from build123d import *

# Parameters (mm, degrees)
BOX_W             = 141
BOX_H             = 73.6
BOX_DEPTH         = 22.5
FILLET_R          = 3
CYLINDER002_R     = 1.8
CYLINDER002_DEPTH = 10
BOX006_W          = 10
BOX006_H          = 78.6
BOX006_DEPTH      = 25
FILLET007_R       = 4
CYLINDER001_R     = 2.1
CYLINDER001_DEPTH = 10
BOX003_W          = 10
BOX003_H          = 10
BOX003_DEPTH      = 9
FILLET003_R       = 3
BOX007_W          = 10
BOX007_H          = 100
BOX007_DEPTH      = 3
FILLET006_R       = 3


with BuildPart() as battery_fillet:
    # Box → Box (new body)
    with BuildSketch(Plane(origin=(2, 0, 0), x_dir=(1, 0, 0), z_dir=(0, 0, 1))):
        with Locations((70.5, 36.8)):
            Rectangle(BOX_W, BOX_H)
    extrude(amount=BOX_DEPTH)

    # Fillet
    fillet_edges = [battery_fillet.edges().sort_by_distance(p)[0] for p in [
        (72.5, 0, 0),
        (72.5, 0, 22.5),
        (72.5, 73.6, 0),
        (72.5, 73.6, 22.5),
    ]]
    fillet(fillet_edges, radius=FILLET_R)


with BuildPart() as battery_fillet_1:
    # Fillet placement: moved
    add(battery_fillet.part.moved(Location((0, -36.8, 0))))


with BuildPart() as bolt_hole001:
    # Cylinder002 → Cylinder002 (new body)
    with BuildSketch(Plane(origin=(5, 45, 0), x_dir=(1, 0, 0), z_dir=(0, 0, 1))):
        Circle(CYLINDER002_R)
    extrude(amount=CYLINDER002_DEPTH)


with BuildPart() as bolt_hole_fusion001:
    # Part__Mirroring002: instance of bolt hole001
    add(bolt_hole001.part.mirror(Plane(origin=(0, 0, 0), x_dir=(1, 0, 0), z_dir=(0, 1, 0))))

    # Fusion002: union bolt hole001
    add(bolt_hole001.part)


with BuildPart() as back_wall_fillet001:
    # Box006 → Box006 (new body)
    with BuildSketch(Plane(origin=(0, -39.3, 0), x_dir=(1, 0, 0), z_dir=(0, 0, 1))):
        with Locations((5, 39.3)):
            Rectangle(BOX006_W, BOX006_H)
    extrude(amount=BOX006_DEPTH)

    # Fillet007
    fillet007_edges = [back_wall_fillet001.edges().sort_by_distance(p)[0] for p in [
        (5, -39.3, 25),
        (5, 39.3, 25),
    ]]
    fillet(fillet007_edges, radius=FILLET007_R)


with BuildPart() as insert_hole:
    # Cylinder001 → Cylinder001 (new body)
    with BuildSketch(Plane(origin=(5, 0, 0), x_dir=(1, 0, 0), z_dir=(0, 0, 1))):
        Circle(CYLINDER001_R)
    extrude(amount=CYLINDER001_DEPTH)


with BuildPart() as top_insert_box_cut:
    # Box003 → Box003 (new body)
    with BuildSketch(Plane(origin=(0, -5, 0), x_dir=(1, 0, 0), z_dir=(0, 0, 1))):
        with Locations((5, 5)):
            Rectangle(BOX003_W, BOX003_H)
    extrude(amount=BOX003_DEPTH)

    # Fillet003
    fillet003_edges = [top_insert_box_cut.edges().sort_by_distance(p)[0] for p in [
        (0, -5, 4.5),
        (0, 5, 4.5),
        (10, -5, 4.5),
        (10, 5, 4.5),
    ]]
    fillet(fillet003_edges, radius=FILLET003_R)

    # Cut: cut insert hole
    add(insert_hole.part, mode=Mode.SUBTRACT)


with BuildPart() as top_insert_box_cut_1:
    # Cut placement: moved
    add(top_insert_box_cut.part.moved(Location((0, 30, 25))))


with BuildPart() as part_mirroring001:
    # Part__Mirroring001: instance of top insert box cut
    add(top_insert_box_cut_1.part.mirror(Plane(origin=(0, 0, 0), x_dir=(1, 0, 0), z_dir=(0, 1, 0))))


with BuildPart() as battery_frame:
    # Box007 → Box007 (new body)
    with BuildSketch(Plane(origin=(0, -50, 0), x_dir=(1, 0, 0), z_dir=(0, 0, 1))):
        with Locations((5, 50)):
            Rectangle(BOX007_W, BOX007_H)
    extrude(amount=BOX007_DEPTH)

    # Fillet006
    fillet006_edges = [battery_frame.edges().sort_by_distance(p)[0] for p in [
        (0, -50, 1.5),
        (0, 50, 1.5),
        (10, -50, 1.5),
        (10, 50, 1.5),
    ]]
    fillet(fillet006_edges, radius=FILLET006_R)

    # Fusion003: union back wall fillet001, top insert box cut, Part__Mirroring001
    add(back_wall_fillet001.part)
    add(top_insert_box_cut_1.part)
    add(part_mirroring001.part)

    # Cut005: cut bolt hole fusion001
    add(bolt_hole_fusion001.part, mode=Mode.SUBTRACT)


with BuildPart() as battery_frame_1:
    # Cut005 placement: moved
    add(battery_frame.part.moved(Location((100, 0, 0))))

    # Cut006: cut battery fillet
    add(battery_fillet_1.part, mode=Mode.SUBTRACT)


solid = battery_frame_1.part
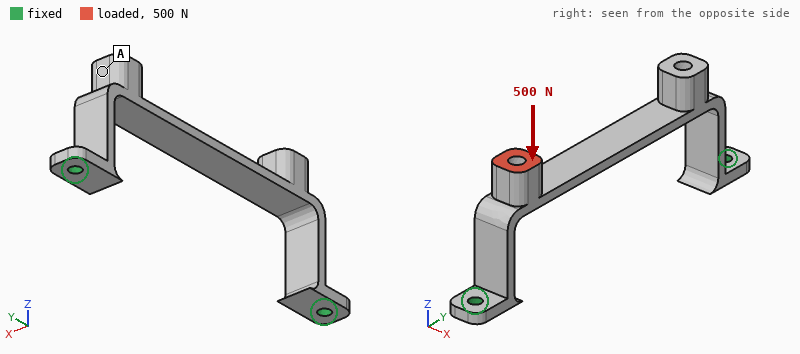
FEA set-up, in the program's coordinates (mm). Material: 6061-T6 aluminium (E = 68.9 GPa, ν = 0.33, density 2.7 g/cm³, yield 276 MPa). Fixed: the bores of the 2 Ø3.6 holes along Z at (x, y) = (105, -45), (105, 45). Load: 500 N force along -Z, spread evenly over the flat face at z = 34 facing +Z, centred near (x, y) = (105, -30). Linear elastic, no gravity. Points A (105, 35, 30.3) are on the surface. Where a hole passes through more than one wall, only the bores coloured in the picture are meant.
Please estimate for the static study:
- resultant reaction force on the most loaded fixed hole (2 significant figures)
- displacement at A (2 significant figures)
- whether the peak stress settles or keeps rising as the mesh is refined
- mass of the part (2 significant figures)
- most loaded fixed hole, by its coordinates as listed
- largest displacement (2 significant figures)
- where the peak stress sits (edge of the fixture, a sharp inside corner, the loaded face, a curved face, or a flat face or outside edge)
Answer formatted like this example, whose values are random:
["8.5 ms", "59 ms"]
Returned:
["470 N", "0.13 mm", "keeps rising", "14 g", "(105, -45)", "0.41 mm", "edge of the fixture"]
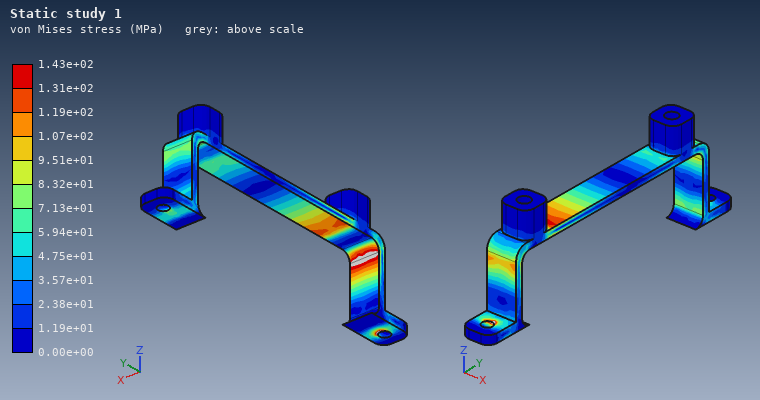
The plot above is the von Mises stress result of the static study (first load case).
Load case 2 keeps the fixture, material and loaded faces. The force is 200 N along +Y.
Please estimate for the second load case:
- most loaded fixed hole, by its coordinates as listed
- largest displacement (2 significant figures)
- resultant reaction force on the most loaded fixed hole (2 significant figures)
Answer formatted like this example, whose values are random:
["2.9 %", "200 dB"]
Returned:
["(105, 45)", "0.45 mm", "160 N"]
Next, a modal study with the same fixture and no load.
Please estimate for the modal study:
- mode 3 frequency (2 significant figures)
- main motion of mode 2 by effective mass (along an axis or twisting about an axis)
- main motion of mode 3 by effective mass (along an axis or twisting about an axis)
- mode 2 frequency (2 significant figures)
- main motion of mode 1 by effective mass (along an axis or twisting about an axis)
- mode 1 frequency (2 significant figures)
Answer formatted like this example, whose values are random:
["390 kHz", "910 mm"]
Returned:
["2000 Hz", "along X", "along Z", "1600 Hz", "along Y", "1500 Hz"]
